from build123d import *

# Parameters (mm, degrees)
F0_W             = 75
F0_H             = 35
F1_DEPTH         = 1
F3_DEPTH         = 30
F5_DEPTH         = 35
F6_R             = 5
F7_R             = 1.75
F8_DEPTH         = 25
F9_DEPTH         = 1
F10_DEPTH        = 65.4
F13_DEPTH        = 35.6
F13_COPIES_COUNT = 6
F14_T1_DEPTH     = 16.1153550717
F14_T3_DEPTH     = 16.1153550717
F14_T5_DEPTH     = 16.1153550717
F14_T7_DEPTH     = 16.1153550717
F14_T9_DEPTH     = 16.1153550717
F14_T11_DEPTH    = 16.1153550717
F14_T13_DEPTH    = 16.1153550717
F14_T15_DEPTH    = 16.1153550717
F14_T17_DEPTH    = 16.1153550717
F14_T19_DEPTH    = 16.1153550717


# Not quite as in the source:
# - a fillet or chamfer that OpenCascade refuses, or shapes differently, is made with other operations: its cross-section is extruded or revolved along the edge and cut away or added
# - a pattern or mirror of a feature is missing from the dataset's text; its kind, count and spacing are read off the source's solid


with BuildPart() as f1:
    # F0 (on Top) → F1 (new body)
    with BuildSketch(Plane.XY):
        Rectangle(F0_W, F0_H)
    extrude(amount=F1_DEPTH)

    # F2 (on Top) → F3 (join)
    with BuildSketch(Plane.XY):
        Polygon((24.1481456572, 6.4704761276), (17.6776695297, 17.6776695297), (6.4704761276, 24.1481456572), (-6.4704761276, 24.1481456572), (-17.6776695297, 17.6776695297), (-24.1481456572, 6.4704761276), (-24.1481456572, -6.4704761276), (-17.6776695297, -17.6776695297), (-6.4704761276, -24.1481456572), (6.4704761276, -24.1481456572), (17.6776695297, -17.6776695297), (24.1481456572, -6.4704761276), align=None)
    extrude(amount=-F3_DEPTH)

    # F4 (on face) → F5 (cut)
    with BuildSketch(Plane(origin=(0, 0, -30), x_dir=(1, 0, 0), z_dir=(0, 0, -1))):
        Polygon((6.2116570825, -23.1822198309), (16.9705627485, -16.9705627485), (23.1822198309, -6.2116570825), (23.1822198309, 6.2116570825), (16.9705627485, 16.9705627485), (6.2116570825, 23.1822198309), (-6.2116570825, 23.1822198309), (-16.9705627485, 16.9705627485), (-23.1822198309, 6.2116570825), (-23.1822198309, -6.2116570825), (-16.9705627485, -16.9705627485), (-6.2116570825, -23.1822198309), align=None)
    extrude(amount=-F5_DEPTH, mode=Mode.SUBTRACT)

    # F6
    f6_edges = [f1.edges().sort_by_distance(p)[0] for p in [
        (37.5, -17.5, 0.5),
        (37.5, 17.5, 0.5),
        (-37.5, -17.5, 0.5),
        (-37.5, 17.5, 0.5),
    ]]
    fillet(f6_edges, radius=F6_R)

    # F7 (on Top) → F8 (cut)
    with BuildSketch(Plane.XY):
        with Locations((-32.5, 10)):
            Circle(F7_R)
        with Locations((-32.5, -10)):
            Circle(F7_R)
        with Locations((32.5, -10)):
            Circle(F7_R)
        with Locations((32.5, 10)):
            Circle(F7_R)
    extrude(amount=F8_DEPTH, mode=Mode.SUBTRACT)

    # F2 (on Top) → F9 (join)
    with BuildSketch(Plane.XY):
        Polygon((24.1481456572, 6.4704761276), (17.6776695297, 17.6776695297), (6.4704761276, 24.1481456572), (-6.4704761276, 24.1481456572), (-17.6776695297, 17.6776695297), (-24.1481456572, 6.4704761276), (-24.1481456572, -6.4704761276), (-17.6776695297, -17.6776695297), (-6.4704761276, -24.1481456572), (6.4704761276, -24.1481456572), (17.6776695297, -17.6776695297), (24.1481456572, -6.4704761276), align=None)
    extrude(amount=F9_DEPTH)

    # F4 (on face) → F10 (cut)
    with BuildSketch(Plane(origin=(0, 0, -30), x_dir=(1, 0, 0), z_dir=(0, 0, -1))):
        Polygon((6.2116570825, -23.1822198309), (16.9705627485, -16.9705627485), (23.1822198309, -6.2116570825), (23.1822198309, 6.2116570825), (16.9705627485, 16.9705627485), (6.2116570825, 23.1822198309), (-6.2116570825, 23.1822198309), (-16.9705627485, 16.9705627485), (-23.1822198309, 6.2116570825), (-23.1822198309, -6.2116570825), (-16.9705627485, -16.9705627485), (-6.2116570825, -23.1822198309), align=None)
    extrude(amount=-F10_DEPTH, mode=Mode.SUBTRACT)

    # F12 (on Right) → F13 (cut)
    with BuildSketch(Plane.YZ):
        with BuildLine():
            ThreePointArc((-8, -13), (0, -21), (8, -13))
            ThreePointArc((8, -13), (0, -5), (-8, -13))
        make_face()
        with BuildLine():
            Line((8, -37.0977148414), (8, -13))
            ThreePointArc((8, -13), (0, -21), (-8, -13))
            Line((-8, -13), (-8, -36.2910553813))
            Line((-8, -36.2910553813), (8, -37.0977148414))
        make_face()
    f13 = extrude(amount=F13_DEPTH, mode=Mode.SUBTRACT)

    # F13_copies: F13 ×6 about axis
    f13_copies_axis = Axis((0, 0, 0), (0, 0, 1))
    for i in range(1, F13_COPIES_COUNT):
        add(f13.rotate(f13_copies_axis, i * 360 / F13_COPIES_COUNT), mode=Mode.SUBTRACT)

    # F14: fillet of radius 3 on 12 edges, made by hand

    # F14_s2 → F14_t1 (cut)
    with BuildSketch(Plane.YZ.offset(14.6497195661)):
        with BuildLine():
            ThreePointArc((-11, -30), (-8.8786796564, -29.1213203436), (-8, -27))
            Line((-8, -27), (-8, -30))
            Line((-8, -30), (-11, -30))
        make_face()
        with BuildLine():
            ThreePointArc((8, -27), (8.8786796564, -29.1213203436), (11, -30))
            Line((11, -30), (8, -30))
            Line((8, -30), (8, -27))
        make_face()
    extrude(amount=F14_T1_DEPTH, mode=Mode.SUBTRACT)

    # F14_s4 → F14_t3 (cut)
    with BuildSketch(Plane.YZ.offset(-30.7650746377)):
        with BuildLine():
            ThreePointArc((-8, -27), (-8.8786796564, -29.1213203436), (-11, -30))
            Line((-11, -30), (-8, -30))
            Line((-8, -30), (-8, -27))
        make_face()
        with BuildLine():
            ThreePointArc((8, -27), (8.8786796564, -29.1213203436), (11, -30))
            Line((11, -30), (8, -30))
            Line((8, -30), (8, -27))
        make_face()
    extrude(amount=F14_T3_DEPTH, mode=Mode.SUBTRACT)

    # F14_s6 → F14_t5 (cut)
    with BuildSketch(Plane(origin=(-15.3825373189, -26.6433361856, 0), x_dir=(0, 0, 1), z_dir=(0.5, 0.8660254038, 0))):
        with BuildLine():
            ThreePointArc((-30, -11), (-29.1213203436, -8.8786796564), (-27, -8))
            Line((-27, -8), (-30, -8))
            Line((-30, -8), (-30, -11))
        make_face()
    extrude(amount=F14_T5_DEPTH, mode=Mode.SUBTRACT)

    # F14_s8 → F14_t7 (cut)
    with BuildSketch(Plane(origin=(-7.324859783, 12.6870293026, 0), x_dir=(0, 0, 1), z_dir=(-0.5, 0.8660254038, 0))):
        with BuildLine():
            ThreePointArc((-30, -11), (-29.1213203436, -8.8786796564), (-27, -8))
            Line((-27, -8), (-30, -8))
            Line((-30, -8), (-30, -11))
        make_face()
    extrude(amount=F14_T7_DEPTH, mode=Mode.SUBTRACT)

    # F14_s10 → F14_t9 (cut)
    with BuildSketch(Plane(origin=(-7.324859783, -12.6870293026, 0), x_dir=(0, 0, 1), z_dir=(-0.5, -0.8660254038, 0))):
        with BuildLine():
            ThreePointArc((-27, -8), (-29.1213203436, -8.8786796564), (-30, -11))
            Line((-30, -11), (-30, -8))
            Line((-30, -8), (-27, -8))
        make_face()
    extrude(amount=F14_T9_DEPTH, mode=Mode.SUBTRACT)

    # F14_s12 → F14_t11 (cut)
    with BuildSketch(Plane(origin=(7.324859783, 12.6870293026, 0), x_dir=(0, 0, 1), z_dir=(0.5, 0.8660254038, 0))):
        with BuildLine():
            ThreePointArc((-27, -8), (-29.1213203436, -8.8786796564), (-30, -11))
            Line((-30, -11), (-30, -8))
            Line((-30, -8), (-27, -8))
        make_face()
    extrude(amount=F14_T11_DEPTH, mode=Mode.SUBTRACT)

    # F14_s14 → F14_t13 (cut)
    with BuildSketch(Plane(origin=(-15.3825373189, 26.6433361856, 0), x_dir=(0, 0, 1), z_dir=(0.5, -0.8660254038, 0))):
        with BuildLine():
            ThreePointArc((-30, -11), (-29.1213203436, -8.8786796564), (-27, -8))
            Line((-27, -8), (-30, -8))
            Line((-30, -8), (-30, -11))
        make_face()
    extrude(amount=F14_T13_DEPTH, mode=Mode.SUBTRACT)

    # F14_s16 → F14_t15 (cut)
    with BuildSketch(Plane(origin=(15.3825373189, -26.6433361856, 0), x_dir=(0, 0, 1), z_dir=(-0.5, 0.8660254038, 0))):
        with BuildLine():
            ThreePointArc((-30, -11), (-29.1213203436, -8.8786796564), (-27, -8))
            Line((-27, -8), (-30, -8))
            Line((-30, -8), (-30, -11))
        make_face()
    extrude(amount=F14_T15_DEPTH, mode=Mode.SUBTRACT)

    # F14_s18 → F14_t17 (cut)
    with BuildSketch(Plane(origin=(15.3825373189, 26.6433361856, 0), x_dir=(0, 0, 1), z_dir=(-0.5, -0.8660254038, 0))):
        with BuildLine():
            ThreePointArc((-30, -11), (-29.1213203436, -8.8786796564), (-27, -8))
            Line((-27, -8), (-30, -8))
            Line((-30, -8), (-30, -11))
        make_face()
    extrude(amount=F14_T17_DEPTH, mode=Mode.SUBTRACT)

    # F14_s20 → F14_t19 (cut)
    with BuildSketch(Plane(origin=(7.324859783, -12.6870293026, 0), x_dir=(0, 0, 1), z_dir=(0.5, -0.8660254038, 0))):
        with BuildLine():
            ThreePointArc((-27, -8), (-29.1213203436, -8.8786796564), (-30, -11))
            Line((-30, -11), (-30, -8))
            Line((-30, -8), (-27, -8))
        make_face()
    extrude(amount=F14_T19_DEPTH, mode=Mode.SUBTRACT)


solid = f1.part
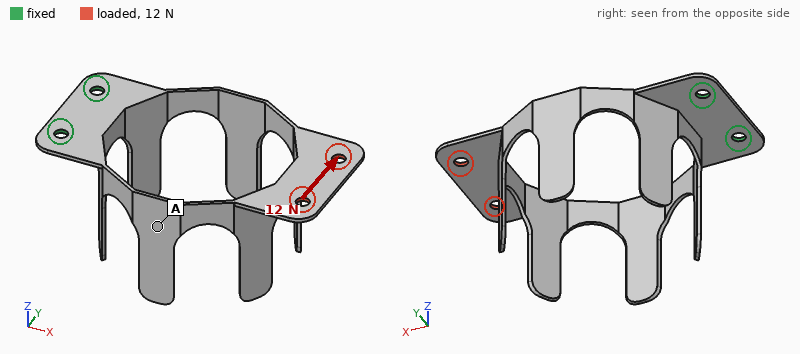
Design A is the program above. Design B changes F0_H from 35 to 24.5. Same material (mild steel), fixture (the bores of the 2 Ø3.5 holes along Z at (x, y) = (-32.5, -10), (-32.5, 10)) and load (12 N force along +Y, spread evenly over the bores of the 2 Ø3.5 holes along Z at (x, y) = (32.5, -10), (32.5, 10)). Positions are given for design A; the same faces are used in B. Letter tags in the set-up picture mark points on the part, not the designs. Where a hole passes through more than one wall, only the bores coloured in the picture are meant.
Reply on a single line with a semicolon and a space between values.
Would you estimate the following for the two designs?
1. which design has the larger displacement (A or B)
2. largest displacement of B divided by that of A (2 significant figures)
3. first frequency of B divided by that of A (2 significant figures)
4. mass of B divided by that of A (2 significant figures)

B; 1.9; 0.93; 0.89
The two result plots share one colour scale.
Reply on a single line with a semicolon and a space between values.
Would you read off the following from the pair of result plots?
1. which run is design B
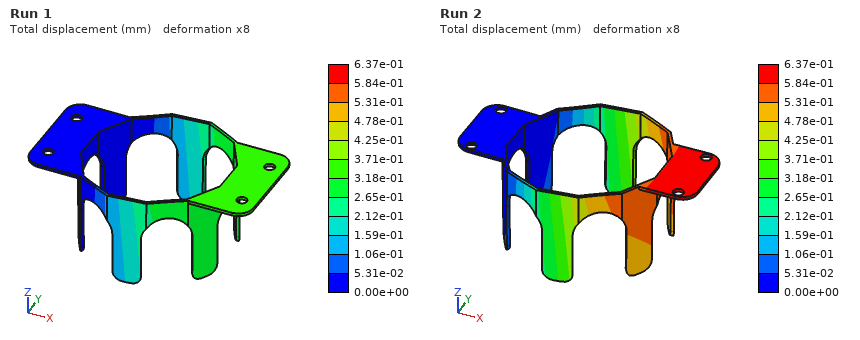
Run 2
